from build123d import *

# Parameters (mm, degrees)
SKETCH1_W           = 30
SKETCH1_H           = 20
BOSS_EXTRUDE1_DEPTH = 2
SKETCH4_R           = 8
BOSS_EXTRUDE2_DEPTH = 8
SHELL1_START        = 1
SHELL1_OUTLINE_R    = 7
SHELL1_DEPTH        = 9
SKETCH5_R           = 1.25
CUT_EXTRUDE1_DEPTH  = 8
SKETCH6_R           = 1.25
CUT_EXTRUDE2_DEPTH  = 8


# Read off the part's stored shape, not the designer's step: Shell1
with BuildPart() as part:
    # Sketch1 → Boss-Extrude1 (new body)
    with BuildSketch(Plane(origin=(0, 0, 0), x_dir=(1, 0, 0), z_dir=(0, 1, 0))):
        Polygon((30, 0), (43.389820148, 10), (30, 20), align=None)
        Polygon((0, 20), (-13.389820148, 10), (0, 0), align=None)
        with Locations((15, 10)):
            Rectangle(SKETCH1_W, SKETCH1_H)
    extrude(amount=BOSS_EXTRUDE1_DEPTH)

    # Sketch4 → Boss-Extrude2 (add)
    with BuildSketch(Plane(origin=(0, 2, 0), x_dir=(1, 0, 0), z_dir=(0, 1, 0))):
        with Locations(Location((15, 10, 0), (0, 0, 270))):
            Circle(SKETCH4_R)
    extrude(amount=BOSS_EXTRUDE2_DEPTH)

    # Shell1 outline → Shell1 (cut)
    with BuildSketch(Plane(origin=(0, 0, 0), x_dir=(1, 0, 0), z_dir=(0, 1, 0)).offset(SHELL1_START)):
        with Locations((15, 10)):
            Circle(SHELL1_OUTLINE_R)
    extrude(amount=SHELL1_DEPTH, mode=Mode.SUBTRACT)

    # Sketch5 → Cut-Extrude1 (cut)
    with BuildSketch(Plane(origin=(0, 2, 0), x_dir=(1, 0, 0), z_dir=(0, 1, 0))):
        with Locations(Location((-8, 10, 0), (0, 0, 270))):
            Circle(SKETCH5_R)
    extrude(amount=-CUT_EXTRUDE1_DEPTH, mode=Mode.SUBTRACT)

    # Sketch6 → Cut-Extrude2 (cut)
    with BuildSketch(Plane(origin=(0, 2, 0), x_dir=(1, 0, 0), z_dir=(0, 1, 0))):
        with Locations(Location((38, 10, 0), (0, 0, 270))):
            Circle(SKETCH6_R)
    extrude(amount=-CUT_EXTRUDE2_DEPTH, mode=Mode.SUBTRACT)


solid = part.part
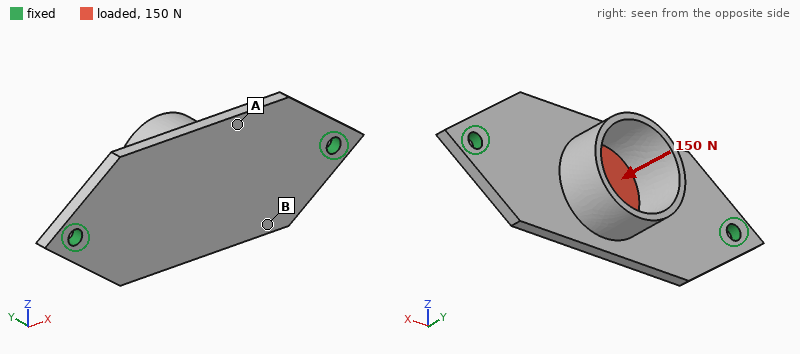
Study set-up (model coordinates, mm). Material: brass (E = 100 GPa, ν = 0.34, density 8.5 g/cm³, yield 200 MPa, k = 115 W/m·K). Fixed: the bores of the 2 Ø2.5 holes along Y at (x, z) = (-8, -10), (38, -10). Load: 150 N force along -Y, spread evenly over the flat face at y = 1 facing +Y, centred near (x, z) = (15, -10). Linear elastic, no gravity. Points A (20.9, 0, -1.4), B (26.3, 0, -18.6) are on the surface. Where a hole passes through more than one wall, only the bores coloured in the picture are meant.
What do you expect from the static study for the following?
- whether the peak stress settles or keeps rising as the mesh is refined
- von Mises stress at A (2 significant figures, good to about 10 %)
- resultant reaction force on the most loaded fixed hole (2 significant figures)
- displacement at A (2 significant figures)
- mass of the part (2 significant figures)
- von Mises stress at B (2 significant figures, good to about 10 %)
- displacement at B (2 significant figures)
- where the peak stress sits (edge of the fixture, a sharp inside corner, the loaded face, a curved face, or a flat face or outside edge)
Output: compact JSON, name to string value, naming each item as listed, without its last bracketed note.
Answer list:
{"whether the peak stress settles or keeps rising as the mesh is refined": "keeps rising", "von Mises stress at A": "34 MPa", "resultant reaction force on the most loaded fixed hole": "82 N", "displacement at A": "49 µm", "mass of the part": "16 g", "von Mises stress at B": "15 MPa", "displacement at B": "35 µm", "where the peak stress sits": "edge of the fixture"}
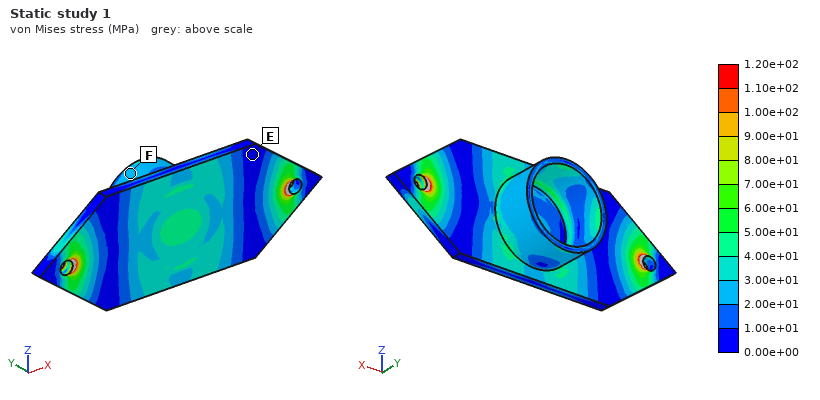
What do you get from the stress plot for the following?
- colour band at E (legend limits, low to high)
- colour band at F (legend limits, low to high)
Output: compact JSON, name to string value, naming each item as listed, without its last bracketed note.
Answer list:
{"colour band at E": "0.00e+00 to 1.00e+01 MPa", "colour band at F": "2.00e+01 to 3.00e+01 MPa"}
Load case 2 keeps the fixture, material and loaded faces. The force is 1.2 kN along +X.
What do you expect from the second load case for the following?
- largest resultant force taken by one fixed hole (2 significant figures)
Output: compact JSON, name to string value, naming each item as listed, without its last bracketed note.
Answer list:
{"largest resultant force taken by one fixed hole": "600 N"}
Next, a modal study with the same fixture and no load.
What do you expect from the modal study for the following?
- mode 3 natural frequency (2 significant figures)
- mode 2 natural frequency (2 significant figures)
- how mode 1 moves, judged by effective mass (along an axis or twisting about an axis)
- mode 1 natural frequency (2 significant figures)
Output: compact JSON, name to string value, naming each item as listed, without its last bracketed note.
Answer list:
{"mode 3 natural frequency": "6800 Hz", "mode 2 natural frequency": "3100 Hz", "how mode 1 moves, judged by effective mass": "along Y", "mode 1 natural frequency": "2800 Hz"}
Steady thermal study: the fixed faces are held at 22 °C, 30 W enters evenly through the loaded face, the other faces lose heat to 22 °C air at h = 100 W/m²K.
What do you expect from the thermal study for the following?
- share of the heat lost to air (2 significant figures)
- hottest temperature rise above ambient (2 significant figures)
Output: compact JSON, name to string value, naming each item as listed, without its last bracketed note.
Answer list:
{"share of the heat lost to air": "35 %", "hottest temperature rise above ambient": "77 K"}
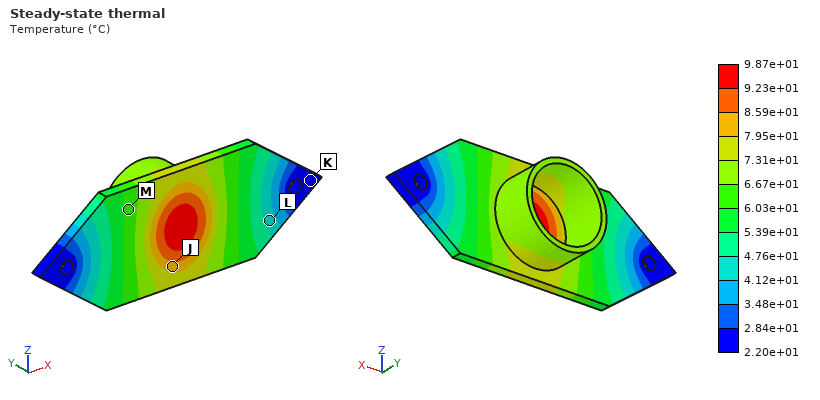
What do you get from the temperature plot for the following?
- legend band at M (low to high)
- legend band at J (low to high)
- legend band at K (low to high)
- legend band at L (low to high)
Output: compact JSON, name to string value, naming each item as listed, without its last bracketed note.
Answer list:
{"legend band at M": "6.03e+01 to 6.67e+01 °C", "legend band at J": "7.95e+01 to 8.59e+01 °C", "legend band at K": "2.20e+01 to 2.84e+01 °C", "legend band at L": "4.12e+01 to 4.76e+01 °C"}
